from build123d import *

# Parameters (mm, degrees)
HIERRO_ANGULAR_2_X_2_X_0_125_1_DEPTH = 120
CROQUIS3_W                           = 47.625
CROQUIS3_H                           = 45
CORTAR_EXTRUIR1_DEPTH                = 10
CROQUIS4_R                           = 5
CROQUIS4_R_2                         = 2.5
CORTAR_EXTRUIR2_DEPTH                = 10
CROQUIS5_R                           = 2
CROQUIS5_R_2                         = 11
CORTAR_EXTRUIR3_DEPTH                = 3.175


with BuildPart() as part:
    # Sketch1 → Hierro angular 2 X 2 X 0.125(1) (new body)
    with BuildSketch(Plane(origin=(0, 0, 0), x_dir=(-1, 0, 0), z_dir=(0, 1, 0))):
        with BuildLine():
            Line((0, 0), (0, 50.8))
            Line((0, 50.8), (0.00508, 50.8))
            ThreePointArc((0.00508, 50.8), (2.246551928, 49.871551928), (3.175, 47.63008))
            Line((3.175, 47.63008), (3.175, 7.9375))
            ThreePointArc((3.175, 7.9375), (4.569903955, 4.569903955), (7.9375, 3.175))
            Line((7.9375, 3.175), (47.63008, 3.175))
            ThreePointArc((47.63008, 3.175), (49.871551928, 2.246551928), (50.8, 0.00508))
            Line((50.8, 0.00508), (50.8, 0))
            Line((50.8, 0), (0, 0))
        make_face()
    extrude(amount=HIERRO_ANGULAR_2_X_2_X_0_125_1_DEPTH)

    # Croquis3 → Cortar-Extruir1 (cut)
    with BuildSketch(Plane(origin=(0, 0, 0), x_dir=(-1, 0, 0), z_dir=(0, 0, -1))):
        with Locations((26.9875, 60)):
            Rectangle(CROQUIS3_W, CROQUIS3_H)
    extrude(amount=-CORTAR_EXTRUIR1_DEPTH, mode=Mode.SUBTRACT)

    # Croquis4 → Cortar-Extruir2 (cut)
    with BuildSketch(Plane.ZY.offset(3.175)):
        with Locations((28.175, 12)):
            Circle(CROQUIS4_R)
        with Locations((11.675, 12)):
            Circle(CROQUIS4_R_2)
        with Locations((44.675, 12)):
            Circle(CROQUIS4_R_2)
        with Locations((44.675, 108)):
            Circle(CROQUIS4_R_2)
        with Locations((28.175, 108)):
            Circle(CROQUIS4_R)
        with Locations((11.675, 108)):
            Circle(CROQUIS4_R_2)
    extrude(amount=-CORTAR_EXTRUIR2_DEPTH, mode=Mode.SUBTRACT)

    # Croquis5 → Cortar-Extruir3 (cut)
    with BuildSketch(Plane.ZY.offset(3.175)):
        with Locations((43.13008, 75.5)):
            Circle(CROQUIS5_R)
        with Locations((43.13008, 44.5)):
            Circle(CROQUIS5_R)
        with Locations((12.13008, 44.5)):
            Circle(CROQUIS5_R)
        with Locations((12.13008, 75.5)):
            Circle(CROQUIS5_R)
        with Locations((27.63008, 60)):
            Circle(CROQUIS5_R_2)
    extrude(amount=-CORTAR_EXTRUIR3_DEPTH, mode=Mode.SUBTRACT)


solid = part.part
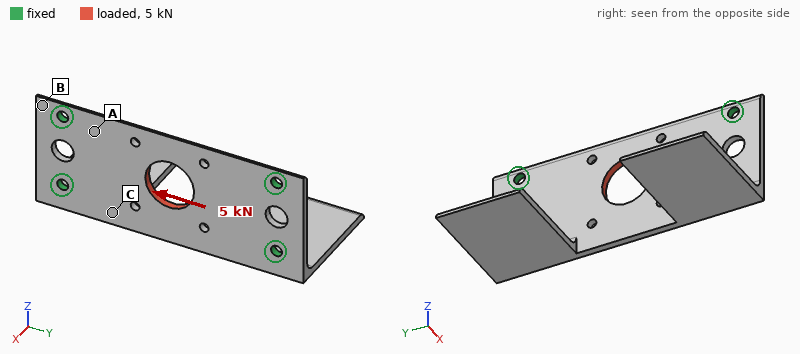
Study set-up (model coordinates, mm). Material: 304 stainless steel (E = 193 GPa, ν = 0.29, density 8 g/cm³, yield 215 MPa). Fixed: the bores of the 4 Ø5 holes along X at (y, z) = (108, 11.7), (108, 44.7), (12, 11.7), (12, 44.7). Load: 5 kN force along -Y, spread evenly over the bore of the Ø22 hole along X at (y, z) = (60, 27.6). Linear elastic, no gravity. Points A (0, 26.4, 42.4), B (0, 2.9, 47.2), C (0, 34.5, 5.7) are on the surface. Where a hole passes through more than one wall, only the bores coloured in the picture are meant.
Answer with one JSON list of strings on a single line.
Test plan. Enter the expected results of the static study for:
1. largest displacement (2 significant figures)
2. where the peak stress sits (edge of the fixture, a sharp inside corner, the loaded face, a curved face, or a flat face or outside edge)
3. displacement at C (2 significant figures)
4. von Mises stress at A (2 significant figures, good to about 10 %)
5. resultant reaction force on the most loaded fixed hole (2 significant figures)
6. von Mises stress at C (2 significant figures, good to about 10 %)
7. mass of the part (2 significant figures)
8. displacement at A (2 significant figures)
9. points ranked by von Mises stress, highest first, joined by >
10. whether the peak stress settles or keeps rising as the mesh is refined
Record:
["5.3 µm", "edge of the fixture", "2.1 µm", "20 MPa", "1.4 kN", "11 MPa", "230 g", "1.7 µm", "A > C > B", "keeps rising"]
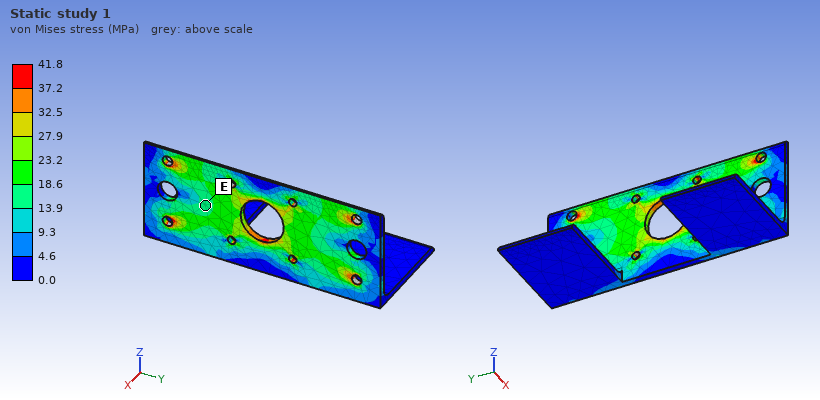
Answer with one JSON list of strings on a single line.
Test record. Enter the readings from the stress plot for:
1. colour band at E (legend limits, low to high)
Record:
["13.9 to 18.6 MPa"]
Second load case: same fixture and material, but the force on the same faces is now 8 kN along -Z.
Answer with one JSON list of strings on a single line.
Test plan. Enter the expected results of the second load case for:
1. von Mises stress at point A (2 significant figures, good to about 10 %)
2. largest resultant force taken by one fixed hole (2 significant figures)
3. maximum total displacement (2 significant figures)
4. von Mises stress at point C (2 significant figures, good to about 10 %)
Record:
["45 MPa", "3.2 kN", "28 µm", "24 MPa"]
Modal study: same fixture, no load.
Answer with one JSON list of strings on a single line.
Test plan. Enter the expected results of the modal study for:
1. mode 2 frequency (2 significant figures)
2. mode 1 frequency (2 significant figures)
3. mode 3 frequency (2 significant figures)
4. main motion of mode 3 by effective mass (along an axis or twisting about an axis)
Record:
["940 Hz", "910 Hz", "1400 Hz", "along X"]
